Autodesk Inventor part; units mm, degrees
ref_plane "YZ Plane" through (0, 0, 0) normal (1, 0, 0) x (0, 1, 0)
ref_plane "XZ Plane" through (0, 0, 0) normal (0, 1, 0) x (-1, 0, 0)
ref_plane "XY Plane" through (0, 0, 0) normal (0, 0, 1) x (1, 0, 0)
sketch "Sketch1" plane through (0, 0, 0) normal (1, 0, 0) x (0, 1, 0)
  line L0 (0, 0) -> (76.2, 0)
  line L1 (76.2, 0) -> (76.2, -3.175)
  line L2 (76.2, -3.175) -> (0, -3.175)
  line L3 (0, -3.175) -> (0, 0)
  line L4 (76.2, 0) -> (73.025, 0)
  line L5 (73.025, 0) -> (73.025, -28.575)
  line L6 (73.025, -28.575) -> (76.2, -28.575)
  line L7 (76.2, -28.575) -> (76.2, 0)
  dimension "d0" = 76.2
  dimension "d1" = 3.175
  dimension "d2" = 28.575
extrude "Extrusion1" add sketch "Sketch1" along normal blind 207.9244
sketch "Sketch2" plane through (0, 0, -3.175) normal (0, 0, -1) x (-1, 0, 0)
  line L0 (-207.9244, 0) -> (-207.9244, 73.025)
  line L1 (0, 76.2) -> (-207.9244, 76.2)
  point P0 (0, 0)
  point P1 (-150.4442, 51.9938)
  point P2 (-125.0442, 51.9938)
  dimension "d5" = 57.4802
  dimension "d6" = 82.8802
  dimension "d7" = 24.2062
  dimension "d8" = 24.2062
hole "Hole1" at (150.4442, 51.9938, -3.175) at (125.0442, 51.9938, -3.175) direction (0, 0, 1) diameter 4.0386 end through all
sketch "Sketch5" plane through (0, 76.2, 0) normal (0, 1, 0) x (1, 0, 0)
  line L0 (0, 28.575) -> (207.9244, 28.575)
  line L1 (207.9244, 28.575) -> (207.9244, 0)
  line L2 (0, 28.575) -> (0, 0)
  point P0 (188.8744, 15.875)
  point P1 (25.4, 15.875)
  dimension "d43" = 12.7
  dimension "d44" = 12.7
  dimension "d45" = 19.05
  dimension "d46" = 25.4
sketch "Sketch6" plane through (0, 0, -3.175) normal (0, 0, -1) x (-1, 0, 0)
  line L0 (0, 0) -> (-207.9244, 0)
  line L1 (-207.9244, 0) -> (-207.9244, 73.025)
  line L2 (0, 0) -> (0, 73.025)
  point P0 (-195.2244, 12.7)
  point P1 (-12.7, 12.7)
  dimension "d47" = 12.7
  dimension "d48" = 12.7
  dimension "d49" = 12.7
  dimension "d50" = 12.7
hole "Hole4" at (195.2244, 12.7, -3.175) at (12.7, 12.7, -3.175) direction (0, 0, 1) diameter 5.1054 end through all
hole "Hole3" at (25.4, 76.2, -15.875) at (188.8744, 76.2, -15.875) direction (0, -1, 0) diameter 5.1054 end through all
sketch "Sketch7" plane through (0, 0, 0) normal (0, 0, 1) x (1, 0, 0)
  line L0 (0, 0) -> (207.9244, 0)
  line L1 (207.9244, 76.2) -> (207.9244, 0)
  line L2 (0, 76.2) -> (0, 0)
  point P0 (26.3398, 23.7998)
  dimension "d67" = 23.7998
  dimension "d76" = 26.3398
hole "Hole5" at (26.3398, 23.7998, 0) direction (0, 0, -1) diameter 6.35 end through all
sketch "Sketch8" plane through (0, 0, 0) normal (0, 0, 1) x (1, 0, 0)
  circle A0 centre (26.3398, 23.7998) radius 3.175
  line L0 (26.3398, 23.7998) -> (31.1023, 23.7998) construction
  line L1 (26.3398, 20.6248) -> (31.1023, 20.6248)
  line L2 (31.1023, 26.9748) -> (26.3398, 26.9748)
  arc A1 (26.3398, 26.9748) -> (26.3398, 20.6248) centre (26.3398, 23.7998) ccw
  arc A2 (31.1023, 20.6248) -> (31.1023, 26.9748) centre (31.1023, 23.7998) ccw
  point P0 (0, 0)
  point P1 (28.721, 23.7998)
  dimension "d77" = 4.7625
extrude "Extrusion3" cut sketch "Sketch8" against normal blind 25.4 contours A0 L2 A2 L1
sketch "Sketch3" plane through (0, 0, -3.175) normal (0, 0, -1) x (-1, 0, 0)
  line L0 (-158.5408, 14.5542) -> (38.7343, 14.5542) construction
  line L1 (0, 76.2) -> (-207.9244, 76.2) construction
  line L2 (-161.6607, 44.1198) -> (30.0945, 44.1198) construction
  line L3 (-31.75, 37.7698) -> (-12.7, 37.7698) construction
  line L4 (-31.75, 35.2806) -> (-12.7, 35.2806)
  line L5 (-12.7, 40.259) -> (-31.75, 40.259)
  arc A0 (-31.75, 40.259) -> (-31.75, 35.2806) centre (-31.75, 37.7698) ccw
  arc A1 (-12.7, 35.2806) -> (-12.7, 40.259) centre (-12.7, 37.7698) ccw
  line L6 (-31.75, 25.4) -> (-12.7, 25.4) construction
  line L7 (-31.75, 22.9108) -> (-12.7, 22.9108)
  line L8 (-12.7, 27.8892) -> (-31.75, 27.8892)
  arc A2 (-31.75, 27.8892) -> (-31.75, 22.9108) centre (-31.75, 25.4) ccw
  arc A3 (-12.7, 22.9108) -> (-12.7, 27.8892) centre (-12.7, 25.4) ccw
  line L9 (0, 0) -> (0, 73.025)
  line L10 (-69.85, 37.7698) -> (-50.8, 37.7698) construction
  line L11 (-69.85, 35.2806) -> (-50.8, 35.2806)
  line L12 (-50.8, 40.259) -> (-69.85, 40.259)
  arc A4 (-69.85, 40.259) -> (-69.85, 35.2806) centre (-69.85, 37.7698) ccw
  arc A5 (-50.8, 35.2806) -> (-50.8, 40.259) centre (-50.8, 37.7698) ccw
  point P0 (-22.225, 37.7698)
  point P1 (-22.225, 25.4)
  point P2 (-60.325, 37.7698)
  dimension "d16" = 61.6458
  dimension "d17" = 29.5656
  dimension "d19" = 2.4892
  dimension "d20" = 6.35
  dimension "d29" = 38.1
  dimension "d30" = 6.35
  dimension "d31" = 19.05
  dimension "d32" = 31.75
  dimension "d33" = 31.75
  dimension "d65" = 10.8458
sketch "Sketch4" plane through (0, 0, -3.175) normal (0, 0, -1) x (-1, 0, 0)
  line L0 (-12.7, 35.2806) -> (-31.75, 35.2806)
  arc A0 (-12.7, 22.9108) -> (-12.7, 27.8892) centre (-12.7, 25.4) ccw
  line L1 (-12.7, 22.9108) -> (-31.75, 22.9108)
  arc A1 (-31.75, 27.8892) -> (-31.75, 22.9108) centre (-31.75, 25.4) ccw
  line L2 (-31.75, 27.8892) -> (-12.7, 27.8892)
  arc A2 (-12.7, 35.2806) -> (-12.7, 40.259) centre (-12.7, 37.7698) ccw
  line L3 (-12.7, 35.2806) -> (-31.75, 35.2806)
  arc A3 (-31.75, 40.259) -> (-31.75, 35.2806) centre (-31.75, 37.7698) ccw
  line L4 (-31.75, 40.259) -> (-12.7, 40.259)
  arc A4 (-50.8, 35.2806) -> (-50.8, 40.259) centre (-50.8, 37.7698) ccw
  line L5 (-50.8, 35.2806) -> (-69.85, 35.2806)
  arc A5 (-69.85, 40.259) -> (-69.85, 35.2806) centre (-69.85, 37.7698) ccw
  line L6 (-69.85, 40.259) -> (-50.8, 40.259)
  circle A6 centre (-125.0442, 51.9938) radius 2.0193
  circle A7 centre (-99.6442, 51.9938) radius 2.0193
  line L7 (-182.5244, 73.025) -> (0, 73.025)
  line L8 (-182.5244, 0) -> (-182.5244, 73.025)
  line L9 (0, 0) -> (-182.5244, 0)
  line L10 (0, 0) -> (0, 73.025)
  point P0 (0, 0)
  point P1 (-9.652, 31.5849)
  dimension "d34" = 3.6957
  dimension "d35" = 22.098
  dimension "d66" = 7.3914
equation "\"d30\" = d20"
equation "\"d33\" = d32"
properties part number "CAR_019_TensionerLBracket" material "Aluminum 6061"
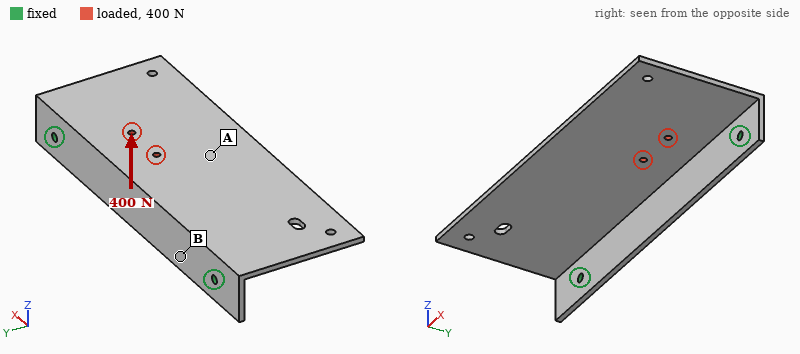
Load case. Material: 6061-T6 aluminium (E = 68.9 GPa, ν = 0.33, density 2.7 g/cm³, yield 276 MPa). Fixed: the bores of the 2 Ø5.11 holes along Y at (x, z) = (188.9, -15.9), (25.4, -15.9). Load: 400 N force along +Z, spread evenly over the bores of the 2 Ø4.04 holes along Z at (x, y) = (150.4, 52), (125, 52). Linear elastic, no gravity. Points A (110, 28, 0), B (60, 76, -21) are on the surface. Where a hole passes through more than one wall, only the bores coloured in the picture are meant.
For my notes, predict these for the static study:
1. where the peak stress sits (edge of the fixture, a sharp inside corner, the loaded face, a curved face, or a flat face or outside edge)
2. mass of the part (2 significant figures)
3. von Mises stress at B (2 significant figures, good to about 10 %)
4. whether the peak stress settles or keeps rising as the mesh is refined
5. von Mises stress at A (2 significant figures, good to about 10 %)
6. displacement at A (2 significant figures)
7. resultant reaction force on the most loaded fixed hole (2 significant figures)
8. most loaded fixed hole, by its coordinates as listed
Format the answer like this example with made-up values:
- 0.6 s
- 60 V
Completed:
- edge of the fixture
- 180 g
- 24 MPa
- keeps rising
- 10 MPa
- 0.68 mm
- 340 N
- (188.9, -15.9)
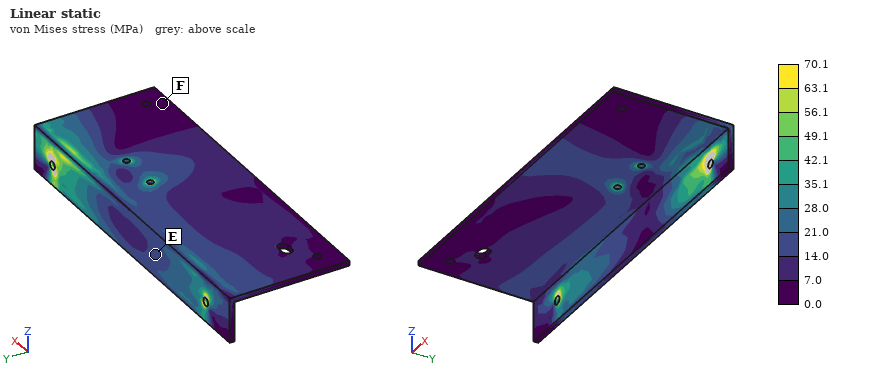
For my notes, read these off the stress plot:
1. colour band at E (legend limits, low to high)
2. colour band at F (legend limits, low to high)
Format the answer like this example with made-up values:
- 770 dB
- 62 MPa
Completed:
- 14.0 to 21.0 MPa
- 0.0 to 7.0 MPa
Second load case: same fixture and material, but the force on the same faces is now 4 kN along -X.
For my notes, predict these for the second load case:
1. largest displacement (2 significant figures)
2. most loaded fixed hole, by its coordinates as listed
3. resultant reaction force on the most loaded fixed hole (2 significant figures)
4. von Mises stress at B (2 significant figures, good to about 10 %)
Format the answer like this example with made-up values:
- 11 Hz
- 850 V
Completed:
- 0.34 mm
- (188.9, -15.9)
- 2.2 kN
- 13 MPa
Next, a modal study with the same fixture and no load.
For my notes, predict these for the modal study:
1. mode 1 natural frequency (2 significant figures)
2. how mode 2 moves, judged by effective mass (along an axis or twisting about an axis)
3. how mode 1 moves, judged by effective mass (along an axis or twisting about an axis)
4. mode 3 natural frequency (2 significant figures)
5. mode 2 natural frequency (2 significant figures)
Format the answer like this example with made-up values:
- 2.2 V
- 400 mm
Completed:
- 270 Hz
- twisting about Y
- along Z
- 860 Hz
- 500 Hz
